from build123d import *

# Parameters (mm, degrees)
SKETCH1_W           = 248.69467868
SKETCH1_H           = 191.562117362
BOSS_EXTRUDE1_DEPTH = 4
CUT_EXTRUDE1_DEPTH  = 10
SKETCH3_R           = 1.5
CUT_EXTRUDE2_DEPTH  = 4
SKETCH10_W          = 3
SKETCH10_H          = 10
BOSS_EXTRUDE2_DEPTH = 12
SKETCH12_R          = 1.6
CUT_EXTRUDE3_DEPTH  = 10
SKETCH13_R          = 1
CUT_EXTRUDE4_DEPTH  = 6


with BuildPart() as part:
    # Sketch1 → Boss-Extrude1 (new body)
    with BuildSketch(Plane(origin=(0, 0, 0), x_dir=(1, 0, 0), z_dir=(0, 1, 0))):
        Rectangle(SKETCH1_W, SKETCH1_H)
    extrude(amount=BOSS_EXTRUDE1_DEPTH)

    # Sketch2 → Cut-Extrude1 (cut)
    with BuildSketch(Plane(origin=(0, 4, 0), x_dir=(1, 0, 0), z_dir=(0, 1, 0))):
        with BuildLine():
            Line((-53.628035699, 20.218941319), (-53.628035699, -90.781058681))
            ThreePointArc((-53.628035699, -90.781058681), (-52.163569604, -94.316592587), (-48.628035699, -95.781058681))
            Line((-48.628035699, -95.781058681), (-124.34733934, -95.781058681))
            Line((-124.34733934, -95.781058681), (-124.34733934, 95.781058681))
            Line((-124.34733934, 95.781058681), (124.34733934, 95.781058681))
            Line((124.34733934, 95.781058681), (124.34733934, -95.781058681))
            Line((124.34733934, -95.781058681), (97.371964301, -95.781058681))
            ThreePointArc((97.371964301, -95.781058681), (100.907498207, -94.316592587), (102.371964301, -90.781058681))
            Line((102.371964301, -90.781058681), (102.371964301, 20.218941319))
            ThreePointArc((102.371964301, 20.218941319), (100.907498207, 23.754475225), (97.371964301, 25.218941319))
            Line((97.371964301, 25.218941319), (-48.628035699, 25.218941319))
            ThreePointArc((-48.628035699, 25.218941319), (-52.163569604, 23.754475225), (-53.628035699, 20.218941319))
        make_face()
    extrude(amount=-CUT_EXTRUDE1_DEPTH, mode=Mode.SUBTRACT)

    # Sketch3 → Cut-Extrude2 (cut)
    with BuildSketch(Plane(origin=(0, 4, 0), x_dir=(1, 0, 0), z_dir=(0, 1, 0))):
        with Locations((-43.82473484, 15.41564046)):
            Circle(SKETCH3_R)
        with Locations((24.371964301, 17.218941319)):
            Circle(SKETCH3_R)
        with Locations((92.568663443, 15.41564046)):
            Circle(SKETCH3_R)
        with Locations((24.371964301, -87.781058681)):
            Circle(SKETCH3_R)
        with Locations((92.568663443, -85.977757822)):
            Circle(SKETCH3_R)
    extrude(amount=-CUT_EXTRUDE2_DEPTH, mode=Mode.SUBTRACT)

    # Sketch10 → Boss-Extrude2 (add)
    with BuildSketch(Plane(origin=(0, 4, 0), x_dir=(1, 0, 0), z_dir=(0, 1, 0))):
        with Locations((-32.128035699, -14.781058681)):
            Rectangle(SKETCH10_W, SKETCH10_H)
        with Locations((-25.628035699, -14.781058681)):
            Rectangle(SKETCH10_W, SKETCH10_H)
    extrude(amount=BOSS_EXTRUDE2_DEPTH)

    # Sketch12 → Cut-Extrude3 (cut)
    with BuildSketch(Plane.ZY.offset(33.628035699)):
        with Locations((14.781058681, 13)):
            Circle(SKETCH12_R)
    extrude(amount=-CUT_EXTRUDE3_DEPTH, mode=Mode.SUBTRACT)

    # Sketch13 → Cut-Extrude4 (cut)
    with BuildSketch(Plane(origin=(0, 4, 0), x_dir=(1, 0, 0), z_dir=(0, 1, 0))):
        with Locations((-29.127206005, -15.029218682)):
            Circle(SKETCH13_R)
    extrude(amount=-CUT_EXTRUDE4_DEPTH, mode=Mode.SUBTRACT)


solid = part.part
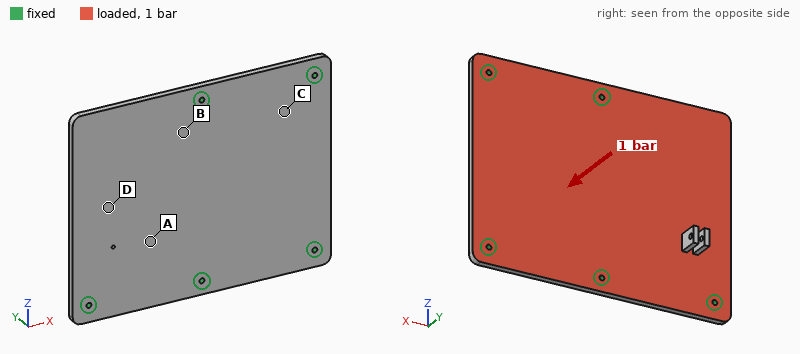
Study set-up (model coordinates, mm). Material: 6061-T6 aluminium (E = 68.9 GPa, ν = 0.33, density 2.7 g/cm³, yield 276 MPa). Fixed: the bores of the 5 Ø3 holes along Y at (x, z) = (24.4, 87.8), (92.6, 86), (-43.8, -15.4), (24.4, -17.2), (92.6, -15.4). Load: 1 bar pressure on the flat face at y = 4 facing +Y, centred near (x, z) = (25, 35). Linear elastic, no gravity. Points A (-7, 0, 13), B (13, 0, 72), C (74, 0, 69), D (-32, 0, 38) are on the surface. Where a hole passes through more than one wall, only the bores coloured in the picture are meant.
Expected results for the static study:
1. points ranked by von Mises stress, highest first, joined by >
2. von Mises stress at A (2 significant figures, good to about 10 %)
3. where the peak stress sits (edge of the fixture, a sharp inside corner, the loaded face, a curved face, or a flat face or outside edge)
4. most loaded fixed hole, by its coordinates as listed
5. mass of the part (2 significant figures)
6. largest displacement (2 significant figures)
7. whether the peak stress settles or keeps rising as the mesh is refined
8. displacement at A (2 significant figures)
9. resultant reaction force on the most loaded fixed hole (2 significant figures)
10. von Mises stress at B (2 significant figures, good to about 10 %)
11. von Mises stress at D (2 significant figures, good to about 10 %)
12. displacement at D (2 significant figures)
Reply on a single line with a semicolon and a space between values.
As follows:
B > D > A > C; 17 MPa; edge of the fixture; (24.4, 87.8); 210 g; 0.83 mm; keeps rising; 0.16 mm; 660 N; 44 MPa; 34 MPa; 0.39 mm
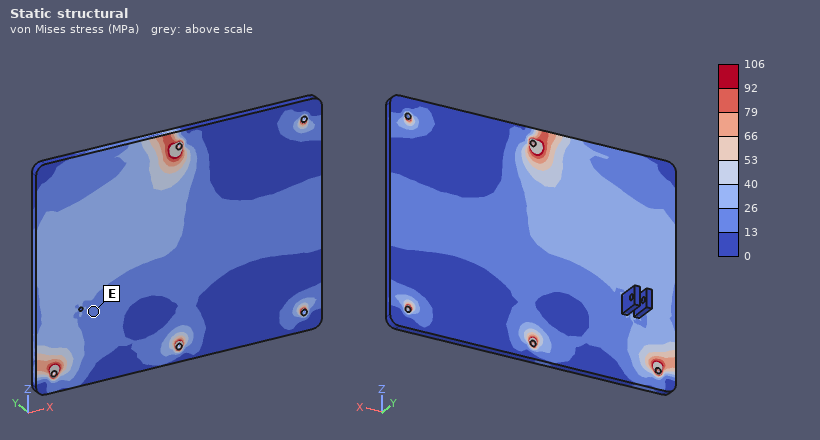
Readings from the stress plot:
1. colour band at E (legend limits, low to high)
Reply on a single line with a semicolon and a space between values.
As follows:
13 to 26 MPa
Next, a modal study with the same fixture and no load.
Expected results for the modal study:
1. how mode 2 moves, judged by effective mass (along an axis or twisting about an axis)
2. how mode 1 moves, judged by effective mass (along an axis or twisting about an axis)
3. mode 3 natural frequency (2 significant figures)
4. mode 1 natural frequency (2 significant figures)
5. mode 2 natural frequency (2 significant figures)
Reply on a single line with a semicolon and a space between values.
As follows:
along Y; along Y; 1900 Hz; 720 Hz; 1500 Hz
